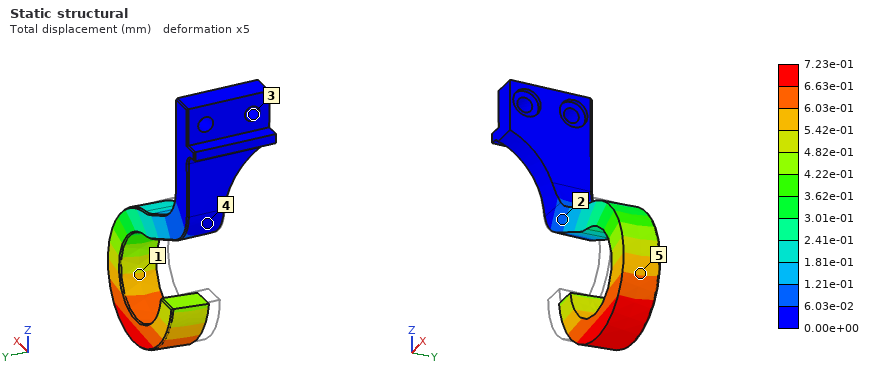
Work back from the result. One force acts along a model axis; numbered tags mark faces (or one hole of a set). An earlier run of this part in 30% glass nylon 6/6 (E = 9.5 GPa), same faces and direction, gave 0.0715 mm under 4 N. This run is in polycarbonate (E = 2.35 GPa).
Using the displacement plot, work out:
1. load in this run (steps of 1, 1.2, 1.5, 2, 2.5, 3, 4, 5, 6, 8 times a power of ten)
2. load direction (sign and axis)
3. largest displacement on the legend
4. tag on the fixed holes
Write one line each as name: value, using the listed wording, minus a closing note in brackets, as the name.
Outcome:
load in this run: 10 N
load direction: +Y
largest displacement on the legend: 7.23e-01 mm
tag on the fixed holes: 3
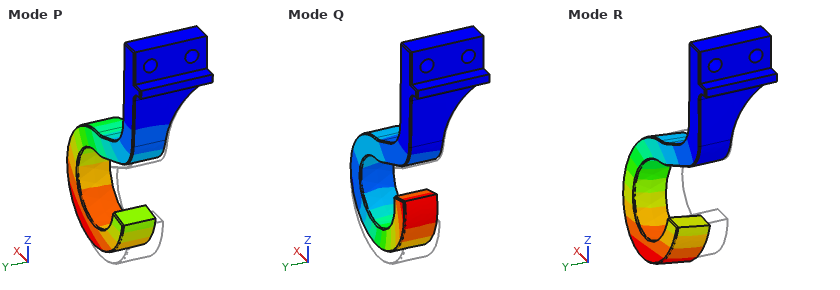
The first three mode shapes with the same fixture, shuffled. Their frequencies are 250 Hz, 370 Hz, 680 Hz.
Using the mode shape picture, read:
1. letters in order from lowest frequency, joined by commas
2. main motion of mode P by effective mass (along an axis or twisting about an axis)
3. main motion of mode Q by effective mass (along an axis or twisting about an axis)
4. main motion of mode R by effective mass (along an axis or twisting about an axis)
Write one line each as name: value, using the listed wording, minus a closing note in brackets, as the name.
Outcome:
letters in order from lowest frequency, joined by commas: P, R, Q
main motion of mode P by effective mass: along X
main motion of mode Q by effective mass: along Z
main motion of mode R by effective mass: along Y
